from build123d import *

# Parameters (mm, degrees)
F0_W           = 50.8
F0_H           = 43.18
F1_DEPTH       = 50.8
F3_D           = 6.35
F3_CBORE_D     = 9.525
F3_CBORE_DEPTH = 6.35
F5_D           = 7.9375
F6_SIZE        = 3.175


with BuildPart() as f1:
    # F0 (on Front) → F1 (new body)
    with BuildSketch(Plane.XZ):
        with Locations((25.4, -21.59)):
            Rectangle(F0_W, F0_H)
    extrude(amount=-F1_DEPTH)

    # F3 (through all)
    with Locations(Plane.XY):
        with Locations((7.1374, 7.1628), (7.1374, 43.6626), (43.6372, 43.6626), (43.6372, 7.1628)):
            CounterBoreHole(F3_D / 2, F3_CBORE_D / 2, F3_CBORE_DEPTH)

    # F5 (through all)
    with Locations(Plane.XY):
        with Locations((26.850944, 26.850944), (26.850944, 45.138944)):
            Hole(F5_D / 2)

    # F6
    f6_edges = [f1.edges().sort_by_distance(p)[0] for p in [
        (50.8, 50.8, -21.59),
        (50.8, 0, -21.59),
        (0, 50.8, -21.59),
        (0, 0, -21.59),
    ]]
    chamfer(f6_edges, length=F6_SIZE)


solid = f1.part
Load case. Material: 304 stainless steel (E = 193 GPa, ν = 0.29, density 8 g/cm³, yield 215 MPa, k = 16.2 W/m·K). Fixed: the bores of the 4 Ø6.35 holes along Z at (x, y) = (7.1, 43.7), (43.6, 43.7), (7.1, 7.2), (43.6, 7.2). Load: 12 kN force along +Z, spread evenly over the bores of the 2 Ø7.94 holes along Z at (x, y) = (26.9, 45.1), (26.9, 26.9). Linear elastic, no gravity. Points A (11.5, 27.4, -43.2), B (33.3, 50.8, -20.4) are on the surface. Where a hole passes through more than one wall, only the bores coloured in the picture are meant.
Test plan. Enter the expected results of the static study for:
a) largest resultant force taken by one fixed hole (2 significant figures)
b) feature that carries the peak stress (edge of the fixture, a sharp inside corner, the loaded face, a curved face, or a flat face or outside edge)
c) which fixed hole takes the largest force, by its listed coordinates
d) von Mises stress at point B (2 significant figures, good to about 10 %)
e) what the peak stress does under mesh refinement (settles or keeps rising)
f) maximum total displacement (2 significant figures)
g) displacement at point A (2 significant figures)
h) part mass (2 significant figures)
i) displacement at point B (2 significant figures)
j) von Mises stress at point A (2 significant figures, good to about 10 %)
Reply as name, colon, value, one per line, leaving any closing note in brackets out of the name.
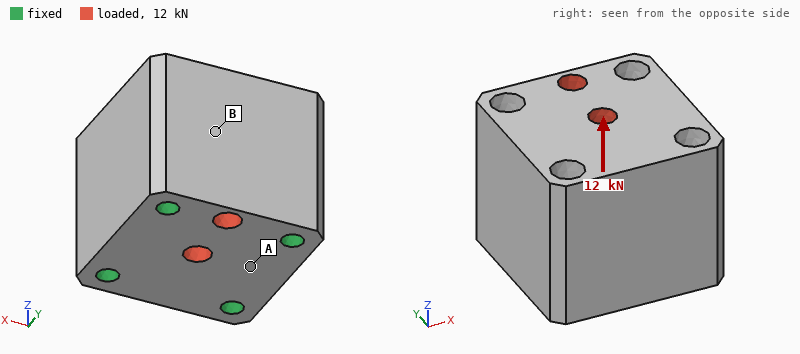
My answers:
largest resultant force taken by one fixed hole: 4.7 kN
feature that carries the peak stress: edge of the fixture
which fixed hole takes the largest force, by its listed coordinates: (43.6, 43.7)
von Mises stress at point B: 13 MPa
what the peak stress does under mesh refinement: keeps rising
maximum total displacement: 1.9 µm
displacement at point A: 0.56 µm
part mass: 800 g
displacement at point B: 0.92 µm
von Mises stress at point A: 3.2 MPa
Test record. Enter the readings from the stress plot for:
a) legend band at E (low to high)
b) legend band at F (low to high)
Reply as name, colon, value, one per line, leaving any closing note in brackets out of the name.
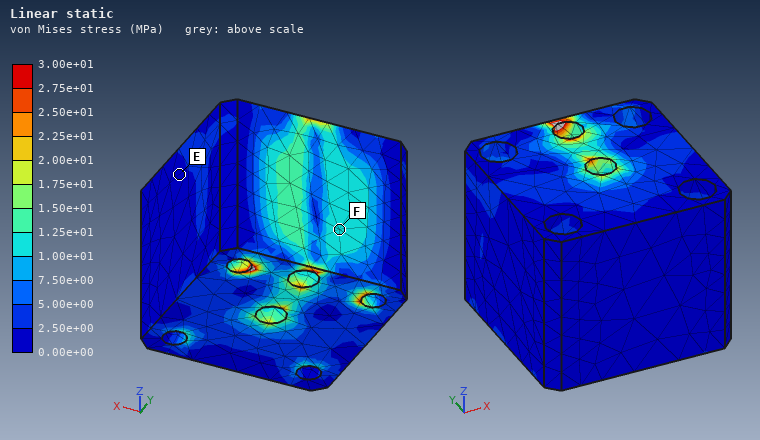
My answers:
legend band at E: 0.00e+00 to 2.50e+00 MPa
legend band at F: 1.00e+01 to 1.25e+01 MPa
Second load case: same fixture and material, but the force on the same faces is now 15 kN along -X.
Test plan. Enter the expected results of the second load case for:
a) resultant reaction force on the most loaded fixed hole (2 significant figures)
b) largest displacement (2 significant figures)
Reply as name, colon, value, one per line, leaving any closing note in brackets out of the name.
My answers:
resultant reaction force on the most loaded fixed hole: 5.7 kN
largest displacement: 0.94 µm
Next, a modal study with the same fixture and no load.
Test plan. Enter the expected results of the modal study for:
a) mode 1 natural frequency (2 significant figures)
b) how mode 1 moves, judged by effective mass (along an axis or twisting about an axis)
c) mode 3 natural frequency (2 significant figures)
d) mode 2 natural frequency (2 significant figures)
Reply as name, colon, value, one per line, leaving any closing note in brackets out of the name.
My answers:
mode 1 natural frequency: 32 kHz
how mode 1 moves, judged by effective mass: along Z
mode 3 natural frequency: 36 kHz
mode 2 natural frequency: 35 kHz
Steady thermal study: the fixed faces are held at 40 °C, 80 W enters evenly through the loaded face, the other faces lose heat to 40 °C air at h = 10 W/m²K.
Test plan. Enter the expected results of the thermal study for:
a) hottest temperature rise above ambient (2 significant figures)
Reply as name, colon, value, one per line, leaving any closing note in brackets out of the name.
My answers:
hottest temperature rise above ambient: 40 K
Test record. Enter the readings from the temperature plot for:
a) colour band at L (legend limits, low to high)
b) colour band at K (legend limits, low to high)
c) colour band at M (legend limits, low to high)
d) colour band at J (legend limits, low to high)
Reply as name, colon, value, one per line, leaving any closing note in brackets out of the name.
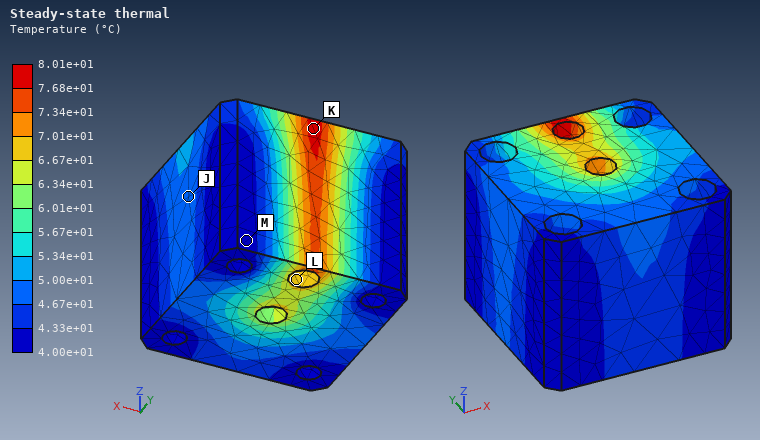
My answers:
colour band at L: 6.67e+01 to 7.01e+01 °C
colour band at K: 7.68e+01 to 8.01e+01 °C
colour band at M: 4.00e+01 to 4.33e+01 °C
colour band at J: 4.67e+01 to 5.00e+01 °C
